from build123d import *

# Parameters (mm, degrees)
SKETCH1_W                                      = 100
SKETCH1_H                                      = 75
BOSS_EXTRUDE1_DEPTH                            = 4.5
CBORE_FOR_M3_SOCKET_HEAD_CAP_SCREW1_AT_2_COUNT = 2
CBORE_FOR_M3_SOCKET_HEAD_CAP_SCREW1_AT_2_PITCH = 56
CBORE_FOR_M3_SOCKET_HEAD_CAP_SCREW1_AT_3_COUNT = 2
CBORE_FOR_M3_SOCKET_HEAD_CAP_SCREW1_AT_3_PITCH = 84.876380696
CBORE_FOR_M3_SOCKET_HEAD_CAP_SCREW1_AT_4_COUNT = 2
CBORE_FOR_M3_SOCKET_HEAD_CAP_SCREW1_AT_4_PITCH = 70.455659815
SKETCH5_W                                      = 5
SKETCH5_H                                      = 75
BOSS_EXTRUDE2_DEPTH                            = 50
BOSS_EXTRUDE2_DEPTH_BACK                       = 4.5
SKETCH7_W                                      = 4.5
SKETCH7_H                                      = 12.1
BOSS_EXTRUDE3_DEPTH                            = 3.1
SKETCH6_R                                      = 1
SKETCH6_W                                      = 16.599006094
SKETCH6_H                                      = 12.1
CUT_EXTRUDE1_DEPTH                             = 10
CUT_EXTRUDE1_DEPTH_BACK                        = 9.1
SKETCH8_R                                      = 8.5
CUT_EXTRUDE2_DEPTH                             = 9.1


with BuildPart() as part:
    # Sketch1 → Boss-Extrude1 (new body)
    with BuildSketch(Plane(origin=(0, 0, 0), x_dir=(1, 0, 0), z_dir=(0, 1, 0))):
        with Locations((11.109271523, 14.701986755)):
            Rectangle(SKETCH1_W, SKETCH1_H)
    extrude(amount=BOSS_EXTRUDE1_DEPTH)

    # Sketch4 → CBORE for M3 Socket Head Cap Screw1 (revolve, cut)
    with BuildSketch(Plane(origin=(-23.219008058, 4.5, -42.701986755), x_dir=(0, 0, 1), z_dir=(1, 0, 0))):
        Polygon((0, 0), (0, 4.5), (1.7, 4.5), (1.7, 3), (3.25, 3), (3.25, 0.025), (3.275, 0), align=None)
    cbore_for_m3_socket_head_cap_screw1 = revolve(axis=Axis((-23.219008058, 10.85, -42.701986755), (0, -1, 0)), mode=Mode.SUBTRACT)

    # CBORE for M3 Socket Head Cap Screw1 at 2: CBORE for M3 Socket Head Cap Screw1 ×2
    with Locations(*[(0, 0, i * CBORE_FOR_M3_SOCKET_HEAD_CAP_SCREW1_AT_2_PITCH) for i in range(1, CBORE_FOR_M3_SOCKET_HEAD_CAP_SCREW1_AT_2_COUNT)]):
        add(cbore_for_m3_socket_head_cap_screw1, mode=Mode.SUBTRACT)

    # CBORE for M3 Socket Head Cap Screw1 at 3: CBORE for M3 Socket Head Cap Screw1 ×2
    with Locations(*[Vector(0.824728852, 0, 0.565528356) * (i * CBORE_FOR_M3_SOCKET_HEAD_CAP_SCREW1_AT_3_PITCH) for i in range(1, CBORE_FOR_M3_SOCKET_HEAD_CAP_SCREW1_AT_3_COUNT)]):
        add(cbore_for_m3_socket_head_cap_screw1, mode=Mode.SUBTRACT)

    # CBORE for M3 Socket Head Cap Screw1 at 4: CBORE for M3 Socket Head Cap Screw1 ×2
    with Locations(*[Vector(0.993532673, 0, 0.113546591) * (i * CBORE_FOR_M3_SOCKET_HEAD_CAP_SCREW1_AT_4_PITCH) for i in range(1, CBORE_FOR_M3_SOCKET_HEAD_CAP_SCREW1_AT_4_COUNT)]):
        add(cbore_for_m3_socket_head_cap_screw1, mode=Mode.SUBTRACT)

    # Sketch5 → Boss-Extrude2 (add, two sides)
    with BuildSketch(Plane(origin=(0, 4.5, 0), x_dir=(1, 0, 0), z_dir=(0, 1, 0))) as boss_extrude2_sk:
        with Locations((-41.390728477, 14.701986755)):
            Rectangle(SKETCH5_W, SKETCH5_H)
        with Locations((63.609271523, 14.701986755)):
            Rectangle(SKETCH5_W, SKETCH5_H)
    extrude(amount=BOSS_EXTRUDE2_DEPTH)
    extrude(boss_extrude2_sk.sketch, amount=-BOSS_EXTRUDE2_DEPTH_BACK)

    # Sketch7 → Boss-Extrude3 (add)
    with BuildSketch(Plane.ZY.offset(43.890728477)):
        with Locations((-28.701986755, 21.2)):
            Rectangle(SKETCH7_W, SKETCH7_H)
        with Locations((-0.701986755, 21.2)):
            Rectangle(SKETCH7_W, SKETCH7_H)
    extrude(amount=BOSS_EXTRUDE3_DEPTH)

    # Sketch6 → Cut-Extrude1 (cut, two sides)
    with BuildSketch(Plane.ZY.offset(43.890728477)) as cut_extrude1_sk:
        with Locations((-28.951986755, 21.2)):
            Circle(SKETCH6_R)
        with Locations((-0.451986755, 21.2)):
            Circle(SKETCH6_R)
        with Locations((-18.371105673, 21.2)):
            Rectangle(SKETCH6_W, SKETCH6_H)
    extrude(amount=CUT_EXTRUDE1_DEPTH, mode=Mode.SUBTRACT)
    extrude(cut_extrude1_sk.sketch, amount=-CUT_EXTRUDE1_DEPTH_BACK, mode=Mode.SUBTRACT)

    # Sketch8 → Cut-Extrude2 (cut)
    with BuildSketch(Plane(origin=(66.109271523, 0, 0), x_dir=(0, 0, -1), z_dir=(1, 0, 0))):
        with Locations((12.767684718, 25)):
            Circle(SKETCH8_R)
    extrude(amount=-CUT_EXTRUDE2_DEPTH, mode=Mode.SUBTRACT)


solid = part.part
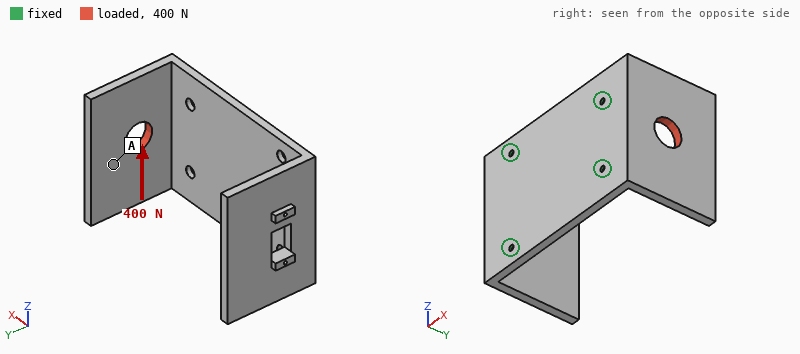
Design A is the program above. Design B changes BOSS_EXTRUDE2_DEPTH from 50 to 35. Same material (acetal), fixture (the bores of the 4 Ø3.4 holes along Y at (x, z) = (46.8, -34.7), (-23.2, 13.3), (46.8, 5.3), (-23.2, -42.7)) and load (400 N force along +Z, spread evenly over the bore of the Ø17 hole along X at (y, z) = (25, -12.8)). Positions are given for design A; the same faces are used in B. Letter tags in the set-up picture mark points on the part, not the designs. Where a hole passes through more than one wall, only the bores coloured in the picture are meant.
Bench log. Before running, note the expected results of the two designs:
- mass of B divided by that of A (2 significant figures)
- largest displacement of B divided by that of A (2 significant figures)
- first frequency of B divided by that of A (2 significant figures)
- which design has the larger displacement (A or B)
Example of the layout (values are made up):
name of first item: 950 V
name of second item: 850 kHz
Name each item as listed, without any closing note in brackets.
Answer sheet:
mass of B divided by that of A: 0.84
largest displacement of B divided by that of A: 0.86
first frequency of B divided by that of A: 1.6
which design has the larger displacement: A
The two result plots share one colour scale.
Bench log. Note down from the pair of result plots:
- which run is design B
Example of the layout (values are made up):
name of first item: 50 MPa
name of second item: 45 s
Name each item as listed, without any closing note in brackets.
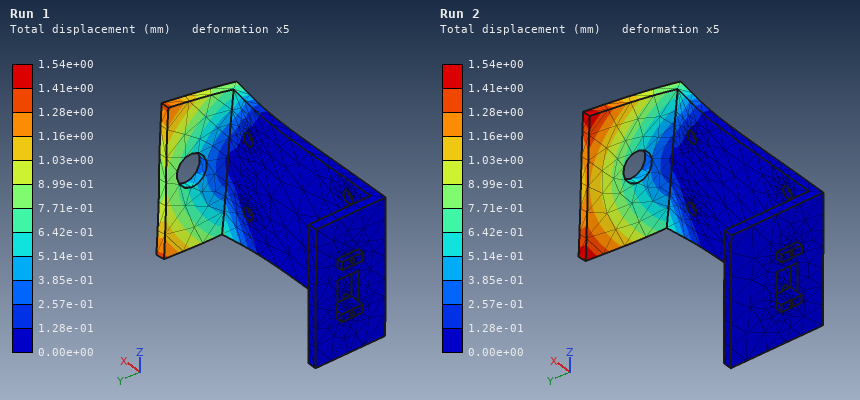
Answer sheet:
which run is design B: Run 1
